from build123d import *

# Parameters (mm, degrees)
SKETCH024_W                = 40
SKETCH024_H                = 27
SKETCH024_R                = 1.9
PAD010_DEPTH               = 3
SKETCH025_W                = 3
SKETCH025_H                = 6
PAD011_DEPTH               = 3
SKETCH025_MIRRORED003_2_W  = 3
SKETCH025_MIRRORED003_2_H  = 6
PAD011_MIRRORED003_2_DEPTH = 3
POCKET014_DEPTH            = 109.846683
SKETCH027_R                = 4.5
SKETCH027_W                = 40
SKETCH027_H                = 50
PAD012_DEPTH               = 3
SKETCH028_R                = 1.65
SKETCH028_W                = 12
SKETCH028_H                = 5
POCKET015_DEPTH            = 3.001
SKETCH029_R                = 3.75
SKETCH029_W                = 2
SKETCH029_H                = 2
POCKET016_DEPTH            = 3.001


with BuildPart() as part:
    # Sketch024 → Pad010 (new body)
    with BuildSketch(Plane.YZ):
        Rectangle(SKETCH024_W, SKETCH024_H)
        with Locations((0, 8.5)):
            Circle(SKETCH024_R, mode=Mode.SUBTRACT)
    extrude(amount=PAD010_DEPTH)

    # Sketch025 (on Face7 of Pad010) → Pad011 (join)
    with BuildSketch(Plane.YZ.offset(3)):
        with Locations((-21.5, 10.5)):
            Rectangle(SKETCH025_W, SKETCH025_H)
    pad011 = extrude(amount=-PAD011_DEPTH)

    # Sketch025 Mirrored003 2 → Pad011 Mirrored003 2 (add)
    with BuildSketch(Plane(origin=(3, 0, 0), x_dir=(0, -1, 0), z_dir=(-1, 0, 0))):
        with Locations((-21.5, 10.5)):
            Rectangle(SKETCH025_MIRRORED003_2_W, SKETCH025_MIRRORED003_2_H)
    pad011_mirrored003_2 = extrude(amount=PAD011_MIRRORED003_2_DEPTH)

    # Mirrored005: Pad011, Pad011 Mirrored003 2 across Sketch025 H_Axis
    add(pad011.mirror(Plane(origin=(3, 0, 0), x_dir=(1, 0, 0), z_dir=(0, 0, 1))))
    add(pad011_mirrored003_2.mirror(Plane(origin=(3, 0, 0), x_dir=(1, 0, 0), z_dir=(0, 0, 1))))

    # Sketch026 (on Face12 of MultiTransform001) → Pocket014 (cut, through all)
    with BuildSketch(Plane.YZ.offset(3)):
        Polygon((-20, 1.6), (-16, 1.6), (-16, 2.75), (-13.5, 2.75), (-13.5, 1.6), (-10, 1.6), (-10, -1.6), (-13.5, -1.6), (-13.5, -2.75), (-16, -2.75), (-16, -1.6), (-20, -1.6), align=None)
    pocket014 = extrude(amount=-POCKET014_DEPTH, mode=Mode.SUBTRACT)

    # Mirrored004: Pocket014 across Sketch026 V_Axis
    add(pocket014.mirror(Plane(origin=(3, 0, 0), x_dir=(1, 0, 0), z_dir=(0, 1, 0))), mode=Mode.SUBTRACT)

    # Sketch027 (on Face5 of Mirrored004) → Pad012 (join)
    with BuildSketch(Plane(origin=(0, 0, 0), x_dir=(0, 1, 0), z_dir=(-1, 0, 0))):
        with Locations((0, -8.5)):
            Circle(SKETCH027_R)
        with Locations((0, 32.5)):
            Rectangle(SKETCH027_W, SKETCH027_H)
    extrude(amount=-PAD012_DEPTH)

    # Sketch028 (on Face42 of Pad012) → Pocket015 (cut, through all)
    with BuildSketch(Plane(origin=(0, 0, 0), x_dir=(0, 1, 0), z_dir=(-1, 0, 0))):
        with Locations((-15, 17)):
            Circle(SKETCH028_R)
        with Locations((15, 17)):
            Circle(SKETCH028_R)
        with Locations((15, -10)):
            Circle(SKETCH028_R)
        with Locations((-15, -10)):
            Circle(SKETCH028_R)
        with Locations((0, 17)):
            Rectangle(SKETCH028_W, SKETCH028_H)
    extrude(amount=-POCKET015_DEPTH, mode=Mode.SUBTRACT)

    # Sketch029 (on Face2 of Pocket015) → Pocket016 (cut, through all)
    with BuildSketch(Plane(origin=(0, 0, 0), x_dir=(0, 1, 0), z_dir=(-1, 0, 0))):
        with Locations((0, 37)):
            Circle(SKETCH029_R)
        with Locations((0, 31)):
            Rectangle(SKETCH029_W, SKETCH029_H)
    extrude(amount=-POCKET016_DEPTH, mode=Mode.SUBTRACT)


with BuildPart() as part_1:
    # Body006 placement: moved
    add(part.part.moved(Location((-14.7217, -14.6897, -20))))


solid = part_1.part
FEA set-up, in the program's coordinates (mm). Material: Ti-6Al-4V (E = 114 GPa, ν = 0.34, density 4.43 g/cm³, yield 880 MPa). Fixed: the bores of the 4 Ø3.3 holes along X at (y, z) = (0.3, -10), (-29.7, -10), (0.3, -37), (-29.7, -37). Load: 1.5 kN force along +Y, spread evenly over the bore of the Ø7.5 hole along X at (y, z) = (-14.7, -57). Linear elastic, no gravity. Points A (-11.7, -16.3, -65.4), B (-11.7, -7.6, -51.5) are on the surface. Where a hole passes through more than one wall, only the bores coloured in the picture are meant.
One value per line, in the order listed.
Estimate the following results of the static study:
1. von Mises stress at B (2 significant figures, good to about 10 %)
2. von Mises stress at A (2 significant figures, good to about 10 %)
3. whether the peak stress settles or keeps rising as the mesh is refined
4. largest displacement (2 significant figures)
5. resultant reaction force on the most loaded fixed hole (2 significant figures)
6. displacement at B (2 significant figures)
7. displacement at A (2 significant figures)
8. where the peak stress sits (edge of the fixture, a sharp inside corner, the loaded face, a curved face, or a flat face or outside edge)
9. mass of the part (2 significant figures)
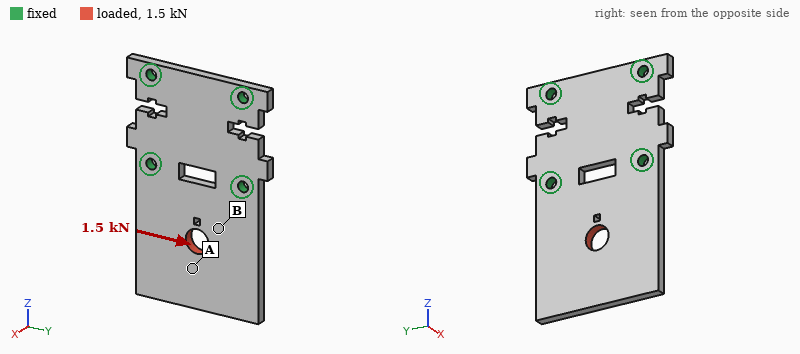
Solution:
30 MPa
11 MPa
keeps rising
16 µm
1.2 kN
7.8 µm
14 µm
edge of the fixture
36 g
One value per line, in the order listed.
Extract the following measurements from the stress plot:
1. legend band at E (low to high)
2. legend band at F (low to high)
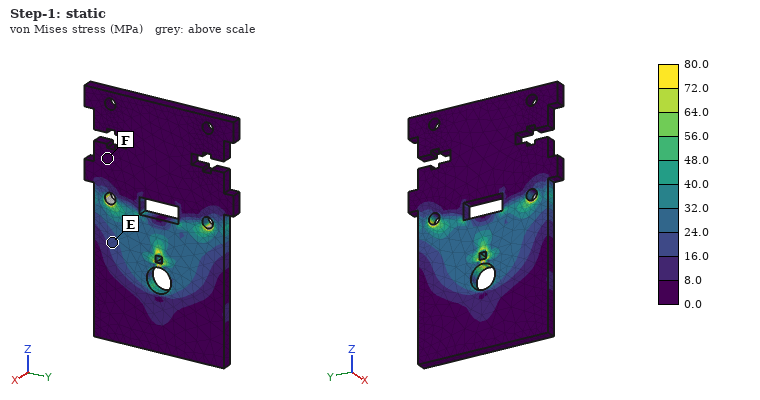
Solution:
16.0 to 24.0 MPa
0.0 to 8.0 MPa
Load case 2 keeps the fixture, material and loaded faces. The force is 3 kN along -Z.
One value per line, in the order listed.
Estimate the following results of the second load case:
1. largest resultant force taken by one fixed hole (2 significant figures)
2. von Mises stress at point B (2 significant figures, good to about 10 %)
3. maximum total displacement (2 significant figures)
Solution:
1.5 kN
33 MPa
10 µm
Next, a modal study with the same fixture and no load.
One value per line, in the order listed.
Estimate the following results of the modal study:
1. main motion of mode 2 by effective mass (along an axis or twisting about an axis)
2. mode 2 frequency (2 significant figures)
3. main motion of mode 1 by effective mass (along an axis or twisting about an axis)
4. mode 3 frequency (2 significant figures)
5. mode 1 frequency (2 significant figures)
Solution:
twisting about Z
3600 Hz
along X
8600 Hz
1400 Hz
